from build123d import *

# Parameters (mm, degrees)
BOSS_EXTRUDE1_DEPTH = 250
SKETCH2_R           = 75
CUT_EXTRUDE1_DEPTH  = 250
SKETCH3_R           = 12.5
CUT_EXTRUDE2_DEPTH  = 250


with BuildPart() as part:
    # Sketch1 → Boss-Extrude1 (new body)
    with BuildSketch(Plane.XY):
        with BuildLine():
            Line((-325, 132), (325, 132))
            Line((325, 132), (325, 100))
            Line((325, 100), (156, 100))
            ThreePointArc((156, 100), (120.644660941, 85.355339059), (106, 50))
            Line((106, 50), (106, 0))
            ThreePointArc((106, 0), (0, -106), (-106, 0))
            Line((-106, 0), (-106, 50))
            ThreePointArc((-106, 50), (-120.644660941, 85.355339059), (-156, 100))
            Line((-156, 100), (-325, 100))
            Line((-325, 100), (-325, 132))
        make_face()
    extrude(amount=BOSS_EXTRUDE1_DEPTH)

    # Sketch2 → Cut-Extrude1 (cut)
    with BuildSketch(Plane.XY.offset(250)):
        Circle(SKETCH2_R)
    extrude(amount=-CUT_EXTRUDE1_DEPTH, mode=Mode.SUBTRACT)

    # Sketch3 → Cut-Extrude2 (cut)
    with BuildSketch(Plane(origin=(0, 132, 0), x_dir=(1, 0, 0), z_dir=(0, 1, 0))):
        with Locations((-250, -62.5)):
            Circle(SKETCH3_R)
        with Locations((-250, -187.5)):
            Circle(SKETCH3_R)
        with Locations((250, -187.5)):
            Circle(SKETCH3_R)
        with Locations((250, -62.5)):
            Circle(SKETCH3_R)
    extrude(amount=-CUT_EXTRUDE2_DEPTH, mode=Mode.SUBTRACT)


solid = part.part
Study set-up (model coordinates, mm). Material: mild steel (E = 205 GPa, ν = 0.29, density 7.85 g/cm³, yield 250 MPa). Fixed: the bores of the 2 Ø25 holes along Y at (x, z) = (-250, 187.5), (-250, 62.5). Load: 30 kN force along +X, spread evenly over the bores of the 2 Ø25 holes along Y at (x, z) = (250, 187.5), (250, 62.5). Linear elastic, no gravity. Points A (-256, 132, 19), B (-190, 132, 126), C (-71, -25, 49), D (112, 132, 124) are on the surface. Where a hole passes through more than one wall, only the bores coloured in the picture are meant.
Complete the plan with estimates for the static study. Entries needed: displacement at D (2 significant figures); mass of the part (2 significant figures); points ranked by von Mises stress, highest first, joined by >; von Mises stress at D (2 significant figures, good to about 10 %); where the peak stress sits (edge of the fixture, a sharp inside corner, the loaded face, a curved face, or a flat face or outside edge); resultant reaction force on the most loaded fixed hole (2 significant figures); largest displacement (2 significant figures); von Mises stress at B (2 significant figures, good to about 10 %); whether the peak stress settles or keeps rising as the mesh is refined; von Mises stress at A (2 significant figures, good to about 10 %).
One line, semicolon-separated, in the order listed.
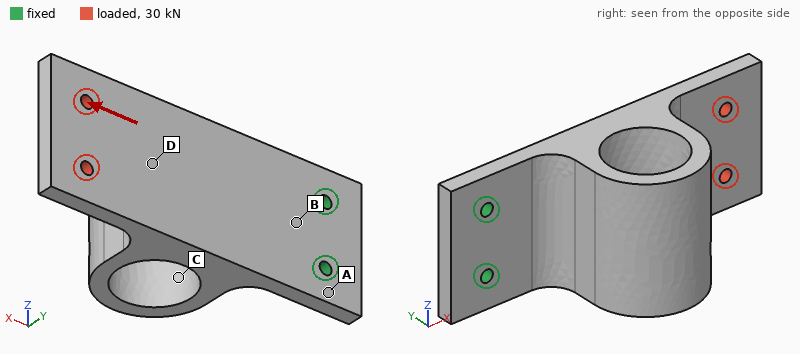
14 µm; 84 kg; D > B > A > C; 4.7 MPa; edge of the fixture; 15 kN; 34 µm; 3.2 MPa; keeps rising; 1.7 MPa
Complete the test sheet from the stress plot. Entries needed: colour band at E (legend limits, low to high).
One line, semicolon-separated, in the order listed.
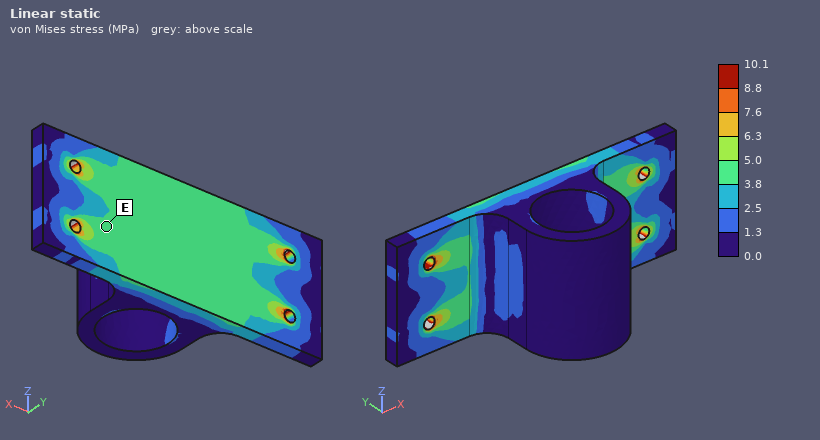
3.8 to 5.0 MPa
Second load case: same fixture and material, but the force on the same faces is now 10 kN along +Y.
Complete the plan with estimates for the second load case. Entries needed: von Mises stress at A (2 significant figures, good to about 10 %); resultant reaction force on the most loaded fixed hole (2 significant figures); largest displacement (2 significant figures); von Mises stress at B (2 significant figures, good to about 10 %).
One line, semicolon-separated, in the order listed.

37 MPa; 5.0 kN; 2.2 mm; 91 MPa
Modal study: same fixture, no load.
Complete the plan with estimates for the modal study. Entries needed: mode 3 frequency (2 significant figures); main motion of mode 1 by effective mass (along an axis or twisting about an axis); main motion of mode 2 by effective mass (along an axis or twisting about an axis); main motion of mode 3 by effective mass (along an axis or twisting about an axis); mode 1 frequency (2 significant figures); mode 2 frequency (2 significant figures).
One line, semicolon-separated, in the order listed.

440 Hz; along Y; along Z; along Z; 72 Hz; 300 Hz
